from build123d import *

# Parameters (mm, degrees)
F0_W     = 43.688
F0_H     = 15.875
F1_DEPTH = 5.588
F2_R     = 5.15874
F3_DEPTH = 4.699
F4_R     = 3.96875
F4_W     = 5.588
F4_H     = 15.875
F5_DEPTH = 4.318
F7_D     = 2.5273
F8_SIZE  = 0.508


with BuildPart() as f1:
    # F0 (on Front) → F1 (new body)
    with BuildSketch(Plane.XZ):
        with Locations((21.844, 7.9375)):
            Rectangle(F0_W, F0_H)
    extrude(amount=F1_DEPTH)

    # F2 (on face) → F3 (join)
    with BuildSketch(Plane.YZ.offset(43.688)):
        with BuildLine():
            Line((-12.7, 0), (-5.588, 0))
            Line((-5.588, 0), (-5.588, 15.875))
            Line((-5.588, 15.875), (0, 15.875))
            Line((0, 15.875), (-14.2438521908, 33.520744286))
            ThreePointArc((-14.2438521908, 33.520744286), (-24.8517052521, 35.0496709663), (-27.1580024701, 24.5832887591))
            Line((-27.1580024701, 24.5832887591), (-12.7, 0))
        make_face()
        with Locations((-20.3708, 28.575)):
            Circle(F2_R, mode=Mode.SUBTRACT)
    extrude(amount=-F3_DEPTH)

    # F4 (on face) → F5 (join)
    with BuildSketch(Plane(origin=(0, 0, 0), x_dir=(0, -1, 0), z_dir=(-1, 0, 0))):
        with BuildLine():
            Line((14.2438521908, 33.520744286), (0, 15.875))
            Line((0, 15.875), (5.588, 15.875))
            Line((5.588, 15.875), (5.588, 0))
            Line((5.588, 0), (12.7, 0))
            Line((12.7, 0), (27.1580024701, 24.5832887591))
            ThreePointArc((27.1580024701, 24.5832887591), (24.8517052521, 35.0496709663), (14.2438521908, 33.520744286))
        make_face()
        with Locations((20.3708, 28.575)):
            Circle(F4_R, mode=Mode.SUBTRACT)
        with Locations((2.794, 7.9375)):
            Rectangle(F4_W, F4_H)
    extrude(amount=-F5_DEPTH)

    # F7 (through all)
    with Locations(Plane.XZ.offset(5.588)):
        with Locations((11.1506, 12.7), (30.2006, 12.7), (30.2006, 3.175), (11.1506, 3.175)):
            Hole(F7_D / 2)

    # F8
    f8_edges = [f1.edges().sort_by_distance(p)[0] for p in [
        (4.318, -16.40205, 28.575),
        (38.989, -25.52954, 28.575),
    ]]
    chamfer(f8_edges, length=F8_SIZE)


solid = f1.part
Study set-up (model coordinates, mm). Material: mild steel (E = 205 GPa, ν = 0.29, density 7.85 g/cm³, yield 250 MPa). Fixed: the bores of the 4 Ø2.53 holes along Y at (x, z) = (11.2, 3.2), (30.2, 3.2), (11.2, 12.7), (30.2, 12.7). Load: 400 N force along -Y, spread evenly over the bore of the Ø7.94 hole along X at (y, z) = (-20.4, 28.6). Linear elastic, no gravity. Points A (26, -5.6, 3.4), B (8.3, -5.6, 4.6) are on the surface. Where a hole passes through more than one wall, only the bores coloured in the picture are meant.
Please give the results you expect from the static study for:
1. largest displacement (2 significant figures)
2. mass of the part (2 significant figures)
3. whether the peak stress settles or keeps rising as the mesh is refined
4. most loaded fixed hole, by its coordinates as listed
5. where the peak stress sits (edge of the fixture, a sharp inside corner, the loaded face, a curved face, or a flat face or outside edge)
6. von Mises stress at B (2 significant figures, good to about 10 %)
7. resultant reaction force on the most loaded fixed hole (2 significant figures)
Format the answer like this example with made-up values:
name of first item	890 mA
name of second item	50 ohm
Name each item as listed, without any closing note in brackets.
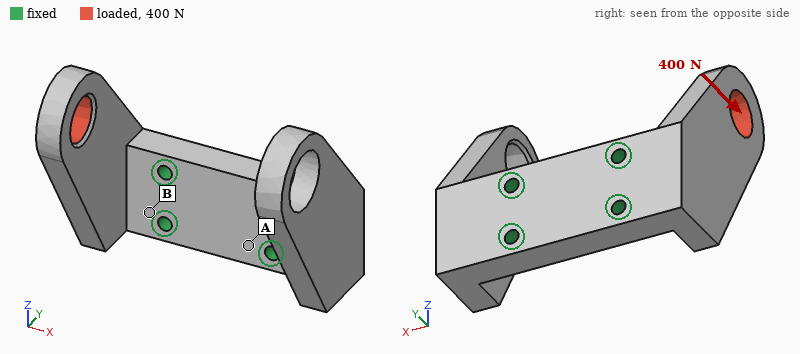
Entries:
largest displacement	40 µm
mass of the part	64 g
whether the peak stress settles or keeps rising as the mesh is refined	keeps rising
most loaded fixed hole, by its coordinates as listed	(11.2, 12.7)
where the peak stress sits	edge of the fixture
von Mises stress at B	52 MPa
resultant reaction force on the most loaded fixed hole	850 N
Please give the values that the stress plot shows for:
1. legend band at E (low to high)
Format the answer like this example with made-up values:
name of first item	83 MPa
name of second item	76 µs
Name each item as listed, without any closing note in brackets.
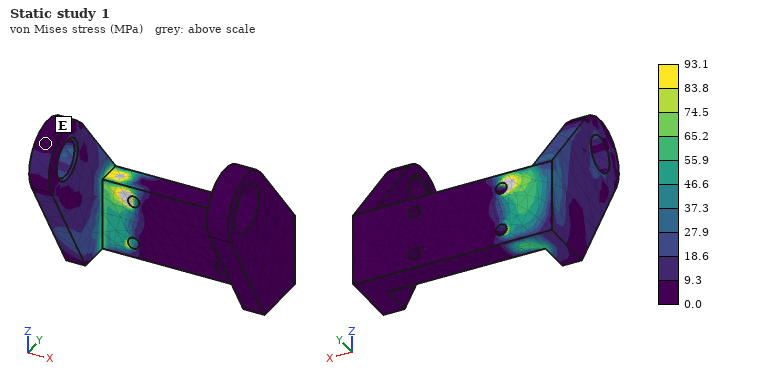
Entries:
legend band at E	0.0 to 9.3 MPa
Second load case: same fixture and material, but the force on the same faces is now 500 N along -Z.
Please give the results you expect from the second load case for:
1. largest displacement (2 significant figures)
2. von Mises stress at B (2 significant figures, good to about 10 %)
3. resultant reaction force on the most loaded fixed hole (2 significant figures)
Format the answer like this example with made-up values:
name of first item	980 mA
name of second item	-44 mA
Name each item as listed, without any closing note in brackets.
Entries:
largest displacement	35 µm
von Mises stress at B	63 MPa
resultant reaction force on the most loaded fixed hole	820 N
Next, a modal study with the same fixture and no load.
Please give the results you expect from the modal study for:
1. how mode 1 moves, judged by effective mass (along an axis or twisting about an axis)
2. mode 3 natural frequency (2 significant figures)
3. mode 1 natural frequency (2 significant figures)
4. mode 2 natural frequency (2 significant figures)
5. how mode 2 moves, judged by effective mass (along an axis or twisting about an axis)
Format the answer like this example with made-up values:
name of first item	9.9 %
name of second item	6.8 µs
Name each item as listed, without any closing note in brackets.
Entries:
how mode 1 moves, judged by effective mass	along X
mode 3 natural frequency	5800 Hz
mode 1 natural frequency	3700 Hz
mode 2 natural frequency	3900 Hz
how mode 2 moves, judged by effective mass	along X
